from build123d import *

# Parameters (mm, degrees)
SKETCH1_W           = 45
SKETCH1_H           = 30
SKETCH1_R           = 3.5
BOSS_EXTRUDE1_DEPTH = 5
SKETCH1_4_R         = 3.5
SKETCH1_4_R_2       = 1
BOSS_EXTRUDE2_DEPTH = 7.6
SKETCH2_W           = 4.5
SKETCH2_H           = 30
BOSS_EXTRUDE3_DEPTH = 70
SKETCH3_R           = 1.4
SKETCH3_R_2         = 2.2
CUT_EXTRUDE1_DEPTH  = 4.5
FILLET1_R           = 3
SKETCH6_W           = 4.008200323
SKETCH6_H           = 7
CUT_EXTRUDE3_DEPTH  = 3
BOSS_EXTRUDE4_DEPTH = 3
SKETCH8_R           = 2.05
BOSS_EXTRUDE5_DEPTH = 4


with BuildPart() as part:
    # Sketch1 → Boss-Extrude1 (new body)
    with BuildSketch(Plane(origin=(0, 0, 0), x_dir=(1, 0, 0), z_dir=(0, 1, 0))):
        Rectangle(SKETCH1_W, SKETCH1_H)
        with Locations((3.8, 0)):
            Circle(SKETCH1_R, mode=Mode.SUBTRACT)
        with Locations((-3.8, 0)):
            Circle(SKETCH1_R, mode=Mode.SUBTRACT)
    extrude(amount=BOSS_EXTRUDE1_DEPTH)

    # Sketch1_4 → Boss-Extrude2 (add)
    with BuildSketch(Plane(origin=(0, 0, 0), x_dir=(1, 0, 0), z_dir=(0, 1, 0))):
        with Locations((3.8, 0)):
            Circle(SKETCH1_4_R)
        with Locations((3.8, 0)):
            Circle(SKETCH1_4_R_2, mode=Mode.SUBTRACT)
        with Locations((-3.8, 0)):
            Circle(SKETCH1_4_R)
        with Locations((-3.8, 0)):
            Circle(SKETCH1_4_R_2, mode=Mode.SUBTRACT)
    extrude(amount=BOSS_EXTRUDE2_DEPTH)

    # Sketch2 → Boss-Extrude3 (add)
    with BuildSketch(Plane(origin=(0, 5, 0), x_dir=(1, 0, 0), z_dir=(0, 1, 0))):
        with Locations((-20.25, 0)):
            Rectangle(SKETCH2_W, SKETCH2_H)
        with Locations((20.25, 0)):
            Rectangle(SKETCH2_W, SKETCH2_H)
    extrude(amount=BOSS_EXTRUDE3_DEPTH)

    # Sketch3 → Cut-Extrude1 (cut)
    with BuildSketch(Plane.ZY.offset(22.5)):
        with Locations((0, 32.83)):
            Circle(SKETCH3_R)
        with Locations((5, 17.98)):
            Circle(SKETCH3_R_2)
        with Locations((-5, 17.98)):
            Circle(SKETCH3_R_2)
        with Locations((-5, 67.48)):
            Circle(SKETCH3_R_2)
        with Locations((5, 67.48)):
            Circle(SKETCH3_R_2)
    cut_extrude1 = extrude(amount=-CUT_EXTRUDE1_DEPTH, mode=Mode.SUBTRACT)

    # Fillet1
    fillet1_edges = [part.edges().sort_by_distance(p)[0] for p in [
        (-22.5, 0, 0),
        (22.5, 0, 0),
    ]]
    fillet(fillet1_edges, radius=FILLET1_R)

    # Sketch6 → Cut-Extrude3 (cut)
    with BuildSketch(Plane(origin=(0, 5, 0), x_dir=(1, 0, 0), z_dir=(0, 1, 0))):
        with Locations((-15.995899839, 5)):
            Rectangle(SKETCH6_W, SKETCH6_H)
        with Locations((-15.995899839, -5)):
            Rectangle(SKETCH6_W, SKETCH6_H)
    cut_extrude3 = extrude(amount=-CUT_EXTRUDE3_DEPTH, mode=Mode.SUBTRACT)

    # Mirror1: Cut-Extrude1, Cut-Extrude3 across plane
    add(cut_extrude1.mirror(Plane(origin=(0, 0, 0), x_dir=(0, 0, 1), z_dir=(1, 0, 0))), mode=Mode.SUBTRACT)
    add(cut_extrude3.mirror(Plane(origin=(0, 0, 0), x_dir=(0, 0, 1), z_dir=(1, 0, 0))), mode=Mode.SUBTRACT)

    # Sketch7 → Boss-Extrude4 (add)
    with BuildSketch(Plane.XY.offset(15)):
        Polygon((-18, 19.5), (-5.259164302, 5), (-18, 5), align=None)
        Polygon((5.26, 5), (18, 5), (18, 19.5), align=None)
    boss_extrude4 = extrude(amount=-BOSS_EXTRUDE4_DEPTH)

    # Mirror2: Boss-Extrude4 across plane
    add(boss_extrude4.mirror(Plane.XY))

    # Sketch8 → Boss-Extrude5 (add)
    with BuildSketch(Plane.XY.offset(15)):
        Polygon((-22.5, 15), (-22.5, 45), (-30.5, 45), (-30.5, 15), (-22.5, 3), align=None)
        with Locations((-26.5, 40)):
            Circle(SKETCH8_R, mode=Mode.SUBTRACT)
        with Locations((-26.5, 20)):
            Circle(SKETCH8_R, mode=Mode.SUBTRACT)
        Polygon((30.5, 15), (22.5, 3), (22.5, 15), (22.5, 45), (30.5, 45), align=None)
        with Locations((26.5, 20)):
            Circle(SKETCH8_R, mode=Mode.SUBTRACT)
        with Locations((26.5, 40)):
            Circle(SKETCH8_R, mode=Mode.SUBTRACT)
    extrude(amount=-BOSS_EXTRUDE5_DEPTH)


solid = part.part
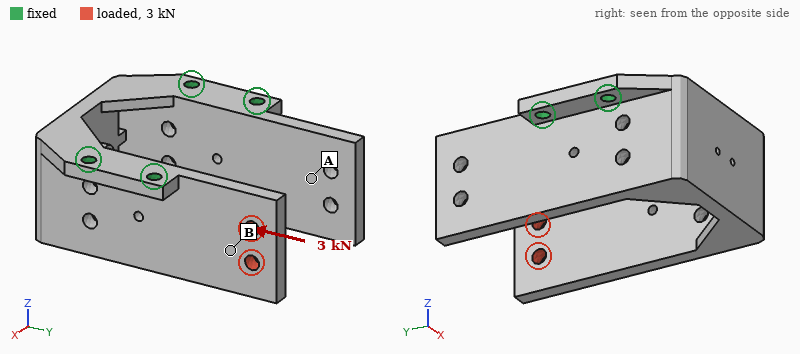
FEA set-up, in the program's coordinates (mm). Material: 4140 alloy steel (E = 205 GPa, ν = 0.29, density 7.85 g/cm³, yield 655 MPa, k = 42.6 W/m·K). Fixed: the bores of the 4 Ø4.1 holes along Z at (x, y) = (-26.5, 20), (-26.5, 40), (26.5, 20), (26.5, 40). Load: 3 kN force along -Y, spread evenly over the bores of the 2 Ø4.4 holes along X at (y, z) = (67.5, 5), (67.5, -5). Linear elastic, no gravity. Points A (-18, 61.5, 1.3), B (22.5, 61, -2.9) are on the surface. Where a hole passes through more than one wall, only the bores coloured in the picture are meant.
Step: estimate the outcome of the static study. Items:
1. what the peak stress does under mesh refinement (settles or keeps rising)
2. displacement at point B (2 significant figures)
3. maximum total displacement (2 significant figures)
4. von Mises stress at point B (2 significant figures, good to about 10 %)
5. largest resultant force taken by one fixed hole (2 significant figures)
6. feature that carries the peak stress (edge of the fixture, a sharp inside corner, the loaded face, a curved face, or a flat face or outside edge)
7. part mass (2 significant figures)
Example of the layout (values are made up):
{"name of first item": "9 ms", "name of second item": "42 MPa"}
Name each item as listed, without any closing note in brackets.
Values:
{"what the peak stress does under mesh refinement": "keeps rising", "displacement at point B": "26 µm", "maximum total displacement": "43 µm", "von Mises stress at point B": "31 MPa", "largest resultant force taken by one fixed hole": "2.2 kN", "feature that carries the peak stress": "edge of the fixture", "part mass": "220 g"}
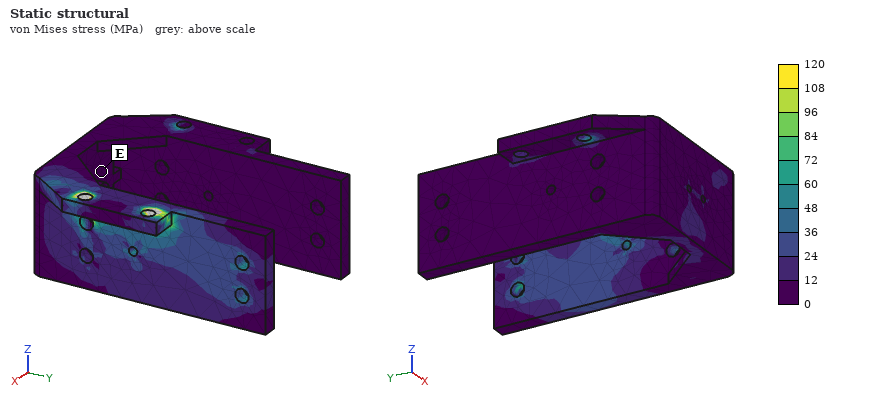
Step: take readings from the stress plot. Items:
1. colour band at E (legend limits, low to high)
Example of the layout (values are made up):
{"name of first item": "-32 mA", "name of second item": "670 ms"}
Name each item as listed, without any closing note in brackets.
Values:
{"colour band at E": "0 to 12 MPa"}
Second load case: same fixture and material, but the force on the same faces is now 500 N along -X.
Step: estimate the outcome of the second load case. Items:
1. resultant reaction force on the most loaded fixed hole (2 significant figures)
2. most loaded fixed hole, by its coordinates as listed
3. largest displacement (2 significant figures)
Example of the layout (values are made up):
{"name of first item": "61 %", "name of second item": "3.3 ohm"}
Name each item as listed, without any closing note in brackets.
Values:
{"resultant reaction force on the most loaded fixed hole": "1.1 kN", "most loaded fixed hole, by its coordinates as listed": "(26.5, 40)", "largest displacement": "0.23 mm"}
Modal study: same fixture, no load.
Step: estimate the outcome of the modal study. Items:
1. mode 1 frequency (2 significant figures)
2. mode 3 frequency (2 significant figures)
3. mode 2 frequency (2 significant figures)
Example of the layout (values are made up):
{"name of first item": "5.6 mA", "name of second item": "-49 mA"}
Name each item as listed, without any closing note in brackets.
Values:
{"mode 1 frequency": "2000 Hz", "mode 3 frequency": "4200 Hz", "mode 2 frequency": "2000 Hz"}
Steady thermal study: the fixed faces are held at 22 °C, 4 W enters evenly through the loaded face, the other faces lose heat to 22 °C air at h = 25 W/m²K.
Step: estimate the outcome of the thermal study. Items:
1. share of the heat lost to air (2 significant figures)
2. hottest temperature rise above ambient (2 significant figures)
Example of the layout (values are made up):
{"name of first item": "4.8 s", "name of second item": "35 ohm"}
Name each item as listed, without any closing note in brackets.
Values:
{"share of the heat lost to air": "34 %", "hottest temperature rise above ambient": "24 K"}
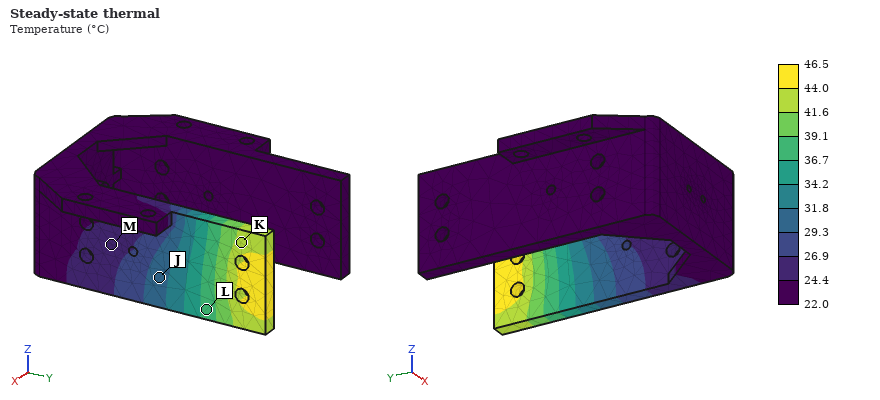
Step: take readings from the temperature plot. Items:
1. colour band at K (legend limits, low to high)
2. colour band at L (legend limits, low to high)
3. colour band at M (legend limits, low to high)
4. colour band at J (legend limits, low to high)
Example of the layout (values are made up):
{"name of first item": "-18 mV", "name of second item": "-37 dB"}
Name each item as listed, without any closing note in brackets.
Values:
{"colour band at K": "41.6 to 44.0 °C", "colour band at L": "36.7 to 39.1 °C", "colour band at M": "24.4 to 26.9 °C", "colour band at J": "29.3 to 31.8 °C"}
